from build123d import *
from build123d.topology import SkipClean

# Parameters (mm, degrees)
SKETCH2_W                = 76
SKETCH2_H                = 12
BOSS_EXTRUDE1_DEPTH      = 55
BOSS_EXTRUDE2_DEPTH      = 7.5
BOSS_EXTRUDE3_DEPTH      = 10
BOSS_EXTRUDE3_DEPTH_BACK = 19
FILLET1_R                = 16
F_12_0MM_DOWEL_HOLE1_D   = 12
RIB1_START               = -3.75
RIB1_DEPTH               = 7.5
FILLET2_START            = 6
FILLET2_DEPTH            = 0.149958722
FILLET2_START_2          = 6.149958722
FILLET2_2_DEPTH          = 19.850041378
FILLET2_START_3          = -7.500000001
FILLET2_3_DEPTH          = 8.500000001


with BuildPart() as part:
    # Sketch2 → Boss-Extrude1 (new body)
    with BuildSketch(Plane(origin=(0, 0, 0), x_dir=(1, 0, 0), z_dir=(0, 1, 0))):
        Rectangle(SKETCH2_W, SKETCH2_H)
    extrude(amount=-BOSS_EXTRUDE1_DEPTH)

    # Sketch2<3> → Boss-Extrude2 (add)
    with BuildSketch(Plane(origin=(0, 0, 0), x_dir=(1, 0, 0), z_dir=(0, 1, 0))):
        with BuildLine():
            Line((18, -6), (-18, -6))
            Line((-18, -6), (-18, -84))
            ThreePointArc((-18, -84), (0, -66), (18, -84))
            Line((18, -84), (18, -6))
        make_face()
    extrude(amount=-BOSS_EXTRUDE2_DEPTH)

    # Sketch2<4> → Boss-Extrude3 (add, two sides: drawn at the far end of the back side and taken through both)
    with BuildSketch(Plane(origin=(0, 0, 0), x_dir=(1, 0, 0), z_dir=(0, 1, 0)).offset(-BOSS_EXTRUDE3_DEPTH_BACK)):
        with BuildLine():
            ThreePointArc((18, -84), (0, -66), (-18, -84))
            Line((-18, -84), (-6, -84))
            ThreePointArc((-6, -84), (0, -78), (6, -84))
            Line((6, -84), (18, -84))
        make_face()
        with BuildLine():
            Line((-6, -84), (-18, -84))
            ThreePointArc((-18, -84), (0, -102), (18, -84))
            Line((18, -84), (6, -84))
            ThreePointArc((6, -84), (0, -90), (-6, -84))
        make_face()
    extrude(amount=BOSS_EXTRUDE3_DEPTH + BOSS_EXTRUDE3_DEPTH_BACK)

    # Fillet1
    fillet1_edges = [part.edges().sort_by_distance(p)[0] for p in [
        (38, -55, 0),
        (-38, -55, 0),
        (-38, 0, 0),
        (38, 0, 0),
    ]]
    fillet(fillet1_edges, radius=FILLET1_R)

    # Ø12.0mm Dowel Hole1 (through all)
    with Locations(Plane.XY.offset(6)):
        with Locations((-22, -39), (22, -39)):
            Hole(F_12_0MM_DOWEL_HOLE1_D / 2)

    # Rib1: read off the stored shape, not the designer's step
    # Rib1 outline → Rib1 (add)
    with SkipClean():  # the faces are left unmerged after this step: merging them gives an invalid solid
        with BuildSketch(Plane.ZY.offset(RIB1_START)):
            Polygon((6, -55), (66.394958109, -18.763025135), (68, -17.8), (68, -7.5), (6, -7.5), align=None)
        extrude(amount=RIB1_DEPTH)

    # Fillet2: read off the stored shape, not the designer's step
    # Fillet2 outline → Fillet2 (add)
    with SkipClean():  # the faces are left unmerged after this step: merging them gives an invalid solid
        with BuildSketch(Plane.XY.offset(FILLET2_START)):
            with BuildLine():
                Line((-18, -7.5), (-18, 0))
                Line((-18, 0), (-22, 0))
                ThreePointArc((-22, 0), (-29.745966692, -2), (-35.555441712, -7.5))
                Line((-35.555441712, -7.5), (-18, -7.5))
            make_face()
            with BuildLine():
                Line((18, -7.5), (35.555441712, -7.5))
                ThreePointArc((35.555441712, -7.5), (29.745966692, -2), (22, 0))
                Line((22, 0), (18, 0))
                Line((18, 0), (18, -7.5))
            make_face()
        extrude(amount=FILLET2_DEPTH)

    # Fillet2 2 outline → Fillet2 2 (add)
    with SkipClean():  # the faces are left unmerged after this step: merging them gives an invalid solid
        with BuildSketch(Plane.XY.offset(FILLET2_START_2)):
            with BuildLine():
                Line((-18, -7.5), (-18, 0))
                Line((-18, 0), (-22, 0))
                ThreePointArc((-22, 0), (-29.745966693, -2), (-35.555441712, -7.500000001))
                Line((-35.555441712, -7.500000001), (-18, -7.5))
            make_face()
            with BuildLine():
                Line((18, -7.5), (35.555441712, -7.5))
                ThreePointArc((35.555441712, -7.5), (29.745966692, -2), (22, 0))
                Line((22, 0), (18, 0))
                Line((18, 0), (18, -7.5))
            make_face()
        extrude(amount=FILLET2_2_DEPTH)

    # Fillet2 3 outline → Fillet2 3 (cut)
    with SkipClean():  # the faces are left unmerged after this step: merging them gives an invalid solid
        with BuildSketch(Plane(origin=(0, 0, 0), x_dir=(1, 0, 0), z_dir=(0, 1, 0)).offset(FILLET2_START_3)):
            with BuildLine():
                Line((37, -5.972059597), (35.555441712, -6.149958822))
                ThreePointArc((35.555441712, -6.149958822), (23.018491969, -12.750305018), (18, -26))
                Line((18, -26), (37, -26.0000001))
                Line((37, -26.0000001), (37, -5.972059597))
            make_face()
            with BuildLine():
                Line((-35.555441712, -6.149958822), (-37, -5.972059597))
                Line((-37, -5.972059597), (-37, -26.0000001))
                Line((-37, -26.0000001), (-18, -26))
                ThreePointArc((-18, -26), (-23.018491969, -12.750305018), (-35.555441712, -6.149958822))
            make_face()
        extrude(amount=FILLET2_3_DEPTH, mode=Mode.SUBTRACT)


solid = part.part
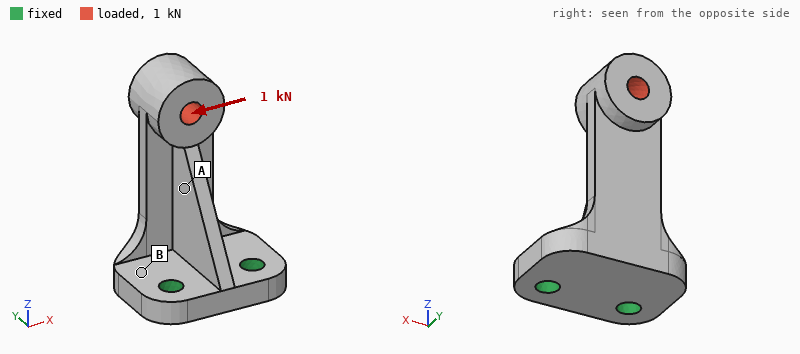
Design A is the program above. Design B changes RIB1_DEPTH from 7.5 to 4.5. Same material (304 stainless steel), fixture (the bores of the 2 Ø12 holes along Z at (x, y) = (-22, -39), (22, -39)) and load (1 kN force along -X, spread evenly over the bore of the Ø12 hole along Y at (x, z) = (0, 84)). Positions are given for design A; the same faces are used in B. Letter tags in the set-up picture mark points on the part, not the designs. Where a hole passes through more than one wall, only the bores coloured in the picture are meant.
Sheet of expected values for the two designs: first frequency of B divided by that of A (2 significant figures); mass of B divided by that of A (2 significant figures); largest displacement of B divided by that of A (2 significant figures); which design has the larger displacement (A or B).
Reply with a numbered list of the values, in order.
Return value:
1. 0.96
2. 0.95
3. 1.1
4. B
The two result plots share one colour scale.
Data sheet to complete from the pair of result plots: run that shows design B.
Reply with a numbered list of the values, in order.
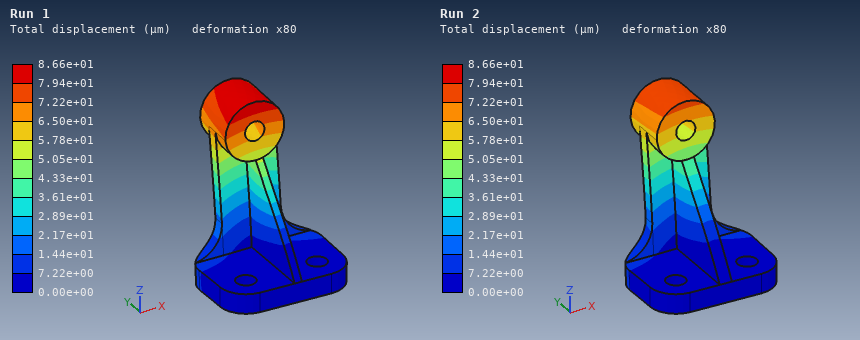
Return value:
1. Run 1
